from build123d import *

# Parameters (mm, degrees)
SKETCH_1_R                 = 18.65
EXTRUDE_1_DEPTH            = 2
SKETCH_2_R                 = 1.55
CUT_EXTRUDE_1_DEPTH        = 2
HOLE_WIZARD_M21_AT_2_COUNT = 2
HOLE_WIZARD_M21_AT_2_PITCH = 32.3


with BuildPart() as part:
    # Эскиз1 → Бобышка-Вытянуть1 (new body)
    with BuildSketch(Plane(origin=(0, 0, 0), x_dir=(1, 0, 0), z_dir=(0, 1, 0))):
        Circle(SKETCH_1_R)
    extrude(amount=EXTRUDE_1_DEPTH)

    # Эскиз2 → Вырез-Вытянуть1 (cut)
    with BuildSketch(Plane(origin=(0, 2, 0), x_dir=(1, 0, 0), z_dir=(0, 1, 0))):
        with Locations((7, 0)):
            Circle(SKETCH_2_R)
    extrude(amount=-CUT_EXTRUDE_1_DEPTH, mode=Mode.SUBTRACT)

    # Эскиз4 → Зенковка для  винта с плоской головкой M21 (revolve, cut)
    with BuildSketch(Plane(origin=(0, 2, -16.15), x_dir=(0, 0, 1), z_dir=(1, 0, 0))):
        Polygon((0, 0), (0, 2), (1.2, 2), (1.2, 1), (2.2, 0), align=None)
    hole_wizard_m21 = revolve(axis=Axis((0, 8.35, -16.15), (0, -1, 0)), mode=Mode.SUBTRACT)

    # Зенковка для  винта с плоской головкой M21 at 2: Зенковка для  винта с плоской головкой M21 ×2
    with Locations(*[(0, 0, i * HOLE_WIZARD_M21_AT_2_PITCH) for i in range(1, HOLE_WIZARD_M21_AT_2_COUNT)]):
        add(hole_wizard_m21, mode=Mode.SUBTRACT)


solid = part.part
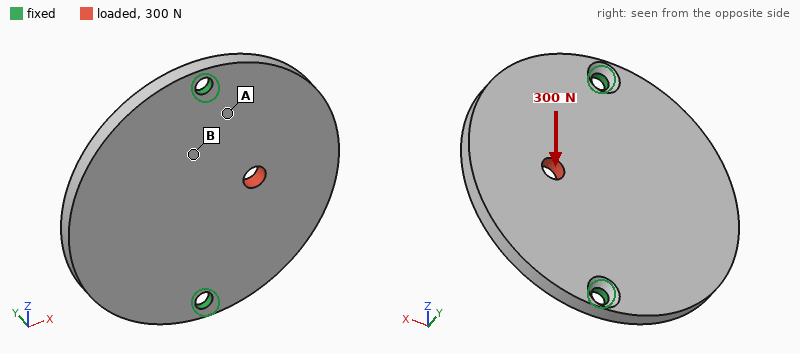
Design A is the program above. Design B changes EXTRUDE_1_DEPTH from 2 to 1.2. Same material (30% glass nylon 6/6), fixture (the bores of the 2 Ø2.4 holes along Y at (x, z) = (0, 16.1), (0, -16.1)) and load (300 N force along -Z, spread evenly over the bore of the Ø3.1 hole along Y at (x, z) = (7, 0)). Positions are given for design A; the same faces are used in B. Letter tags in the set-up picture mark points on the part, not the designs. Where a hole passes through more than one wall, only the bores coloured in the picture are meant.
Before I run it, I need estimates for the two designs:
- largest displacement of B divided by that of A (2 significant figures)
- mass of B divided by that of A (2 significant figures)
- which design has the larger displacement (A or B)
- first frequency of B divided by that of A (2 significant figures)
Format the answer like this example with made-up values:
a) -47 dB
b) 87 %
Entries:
a) 1.5
b) 0.60
c) B
d) 0.77
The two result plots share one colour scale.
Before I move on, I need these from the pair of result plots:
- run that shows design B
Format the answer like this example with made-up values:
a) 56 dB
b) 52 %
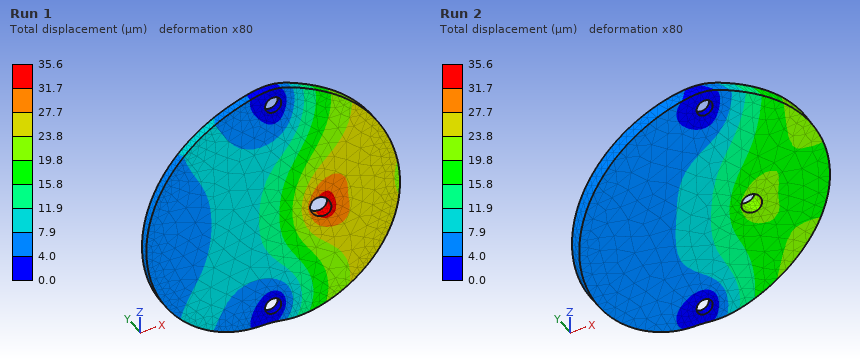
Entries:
a) Run 1
